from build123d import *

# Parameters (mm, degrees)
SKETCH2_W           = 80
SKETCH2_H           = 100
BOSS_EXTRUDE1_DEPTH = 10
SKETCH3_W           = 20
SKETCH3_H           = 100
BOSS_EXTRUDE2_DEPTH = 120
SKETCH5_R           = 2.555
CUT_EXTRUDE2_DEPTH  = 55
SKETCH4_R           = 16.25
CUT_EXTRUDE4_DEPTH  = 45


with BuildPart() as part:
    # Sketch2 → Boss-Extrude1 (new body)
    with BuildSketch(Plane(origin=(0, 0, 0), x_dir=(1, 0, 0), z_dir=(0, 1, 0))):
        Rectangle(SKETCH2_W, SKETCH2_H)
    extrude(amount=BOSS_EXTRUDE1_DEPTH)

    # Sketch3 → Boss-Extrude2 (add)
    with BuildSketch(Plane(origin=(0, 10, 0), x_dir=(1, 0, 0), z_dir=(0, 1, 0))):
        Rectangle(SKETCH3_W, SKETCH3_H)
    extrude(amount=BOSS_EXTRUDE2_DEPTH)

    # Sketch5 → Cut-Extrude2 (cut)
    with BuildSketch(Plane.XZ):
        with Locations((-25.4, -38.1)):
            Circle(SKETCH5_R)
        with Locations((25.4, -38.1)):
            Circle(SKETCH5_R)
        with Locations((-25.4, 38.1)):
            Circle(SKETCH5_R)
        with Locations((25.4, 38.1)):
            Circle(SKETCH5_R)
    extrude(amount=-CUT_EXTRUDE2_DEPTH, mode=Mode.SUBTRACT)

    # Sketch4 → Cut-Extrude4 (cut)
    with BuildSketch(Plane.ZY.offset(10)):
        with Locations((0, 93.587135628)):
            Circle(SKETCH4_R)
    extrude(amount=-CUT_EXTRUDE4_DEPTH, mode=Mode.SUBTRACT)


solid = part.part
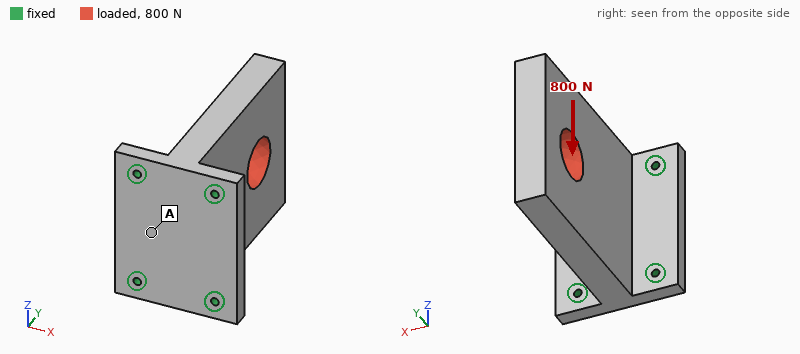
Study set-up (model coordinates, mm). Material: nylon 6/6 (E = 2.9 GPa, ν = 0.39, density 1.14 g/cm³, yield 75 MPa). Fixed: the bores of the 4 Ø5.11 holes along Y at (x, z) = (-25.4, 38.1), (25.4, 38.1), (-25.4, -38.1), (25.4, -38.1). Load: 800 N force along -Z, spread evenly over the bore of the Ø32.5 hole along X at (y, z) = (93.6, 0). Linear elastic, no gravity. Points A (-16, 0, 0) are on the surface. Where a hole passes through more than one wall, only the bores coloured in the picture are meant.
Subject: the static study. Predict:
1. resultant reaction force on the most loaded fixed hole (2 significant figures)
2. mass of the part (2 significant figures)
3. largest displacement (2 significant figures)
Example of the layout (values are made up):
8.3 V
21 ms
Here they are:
520 N
340 g
0.40 mm
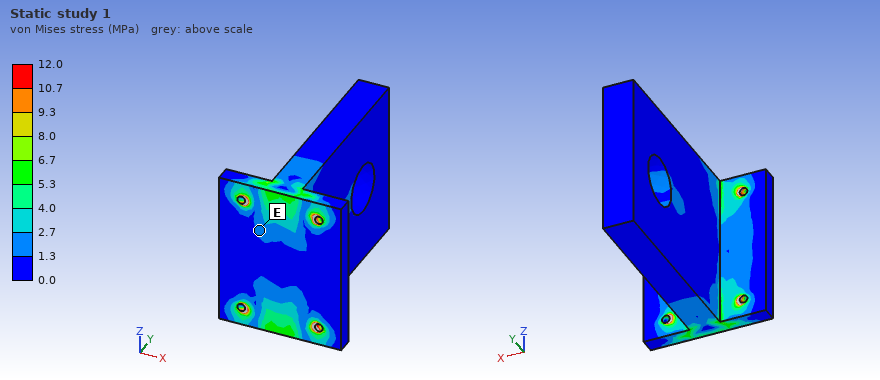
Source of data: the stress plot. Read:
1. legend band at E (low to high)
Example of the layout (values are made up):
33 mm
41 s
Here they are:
1.3 to 2.7 MPa
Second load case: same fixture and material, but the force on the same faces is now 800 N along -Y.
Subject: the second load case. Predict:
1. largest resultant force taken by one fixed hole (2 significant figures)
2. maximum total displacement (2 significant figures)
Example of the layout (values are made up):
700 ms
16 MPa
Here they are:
210 N
56 µm
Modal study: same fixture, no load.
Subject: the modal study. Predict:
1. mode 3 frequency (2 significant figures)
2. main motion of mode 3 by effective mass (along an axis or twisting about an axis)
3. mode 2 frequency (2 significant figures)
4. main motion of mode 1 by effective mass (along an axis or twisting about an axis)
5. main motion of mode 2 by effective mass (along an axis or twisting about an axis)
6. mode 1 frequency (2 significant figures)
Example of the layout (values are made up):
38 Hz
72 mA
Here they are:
770 Hz
twisting about Y
630 Hz
along X
along Z
280 Hz
